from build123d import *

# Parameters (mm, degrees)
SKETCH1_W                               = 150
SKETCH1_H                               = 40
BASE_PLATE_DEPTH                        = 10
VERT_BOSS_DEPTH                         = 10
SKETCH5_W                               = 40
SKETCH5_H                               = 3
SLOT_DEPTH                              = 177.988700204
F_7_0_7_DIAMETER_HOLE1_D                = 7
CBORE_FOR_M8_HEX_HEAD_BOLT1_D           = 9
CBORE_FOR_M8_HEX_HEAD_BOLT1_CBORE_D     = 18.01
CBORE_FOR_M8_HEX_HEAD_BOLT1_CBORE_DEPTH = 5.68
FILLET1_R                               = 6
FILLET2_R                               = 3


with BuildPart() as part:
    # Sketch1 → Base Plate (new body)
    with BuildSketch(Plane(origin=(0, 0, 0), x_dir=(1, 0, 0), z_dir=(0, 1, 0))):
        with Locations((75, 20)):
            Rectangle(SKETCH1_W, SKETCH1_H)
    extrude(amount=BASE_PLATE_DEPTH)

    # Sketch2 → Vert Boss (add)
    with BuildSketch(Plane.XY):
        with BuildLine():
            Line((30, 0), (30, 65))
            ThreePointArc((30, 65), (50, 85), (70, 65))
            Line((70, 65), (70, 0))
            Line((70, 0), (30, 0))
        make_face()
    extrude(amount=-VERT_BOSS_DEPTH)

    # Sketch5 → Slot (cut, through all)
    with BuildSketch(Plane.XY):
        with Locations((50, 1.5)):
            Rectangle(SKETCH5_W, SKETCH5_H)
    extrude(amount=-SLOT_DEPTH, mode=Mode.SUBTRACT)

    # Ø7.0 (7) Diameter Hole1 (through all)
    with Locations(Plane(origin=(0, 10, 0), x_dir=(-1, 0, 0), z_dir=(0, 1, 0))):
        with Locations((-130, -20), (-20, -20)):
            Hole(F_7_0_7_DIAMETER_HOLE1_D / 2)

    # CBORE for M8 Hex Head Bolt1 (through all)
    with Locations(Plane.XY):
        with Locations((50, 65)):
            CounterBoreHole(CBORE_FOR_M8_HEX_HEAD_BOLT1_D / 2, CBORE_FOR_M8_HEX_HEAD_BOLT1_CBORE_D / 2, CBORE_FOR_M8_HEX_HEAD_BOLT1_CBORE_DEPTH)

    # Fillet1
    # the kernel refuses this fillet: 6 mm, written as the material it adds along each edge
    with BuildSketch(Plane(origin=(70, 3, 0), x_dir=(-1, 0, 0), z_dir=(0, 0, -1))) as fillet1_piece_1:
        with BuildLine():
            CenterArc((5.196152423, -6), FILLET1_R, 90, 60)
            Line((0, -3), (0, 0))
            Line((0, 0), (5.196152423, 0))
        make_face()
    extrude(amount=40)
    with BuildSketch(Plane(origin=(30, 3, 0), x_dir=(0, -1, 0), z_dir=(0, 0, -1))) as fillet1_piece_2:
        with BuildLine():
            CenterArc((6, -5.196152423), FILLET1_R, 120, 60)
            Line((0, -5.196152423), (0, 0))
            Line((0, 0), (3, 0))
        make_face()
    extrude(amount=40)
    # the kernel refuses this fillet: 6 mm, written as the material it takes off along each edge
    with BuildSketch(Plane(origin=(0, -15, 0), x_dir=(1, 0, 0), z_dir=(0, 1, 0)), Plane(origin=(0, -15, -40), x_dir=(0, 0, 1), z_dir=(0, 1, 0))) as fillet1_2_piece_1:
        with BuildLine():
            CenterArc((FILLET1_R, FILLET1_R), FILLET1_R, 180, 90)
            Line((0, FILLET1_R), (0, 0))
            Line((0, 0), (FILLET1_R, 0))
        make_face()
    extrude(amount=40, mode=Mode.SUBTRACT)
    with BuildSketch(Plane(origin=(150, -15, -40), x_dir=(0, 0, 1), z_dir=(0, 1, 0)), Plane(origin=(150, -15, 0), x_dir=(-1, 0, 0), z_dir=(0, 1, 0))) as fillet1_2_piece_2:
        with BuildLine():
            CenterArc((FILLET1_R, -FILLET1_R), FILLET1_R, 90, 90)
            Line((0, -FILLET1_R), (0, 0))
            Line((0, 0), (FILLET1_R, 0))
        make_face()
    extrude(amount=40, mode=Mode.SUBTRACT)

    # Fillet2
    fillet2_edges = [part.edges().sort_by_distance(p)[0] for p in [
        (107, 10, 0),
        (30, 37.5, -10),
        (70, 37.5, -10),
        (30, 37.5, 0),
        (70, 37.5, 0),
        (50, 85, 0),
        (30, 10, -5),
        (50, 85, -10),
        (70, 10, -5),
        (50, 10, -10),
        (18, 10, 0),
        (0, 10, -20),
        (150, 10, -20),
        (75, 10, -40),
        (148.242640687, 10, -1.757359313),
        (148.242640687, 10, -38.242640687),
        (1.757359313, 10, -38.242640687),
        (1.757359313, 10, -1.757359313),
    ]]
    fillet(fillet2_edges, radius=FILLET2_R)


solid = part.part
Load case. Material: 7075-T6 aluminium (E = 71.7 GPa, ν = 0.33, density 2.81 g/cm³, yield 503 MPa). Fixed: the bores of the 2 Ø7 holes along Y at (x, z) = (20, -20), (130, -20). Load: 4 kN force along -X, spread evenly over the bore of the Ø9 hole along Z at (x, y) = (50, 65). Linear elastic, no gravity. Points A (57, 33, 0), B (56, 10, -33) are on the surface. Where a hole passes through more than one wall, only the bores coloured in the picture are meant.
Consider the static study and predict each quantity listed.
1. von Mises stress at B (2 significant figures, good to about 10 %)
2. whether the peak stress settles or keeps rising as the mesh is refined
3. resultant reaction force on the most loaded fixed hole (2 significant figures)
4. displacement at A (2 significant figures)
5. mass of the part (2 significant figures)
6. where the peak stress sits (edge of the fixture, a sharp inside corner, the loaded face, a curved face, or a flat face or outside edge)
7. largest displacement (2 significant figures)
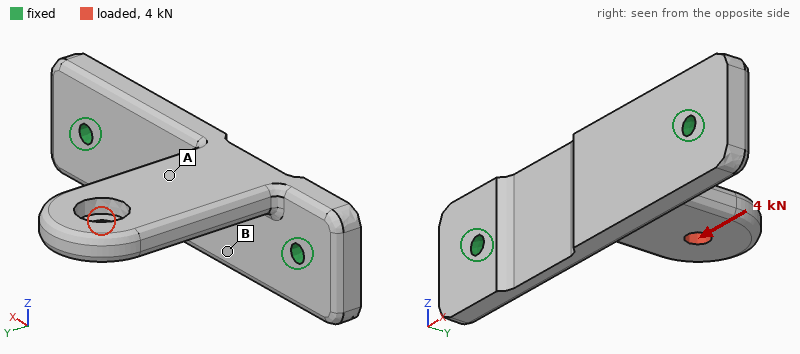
61 MPa
keeps rising
3.3 kN
0.32 mm
220 g
a sharp inside corner
0.80 mm
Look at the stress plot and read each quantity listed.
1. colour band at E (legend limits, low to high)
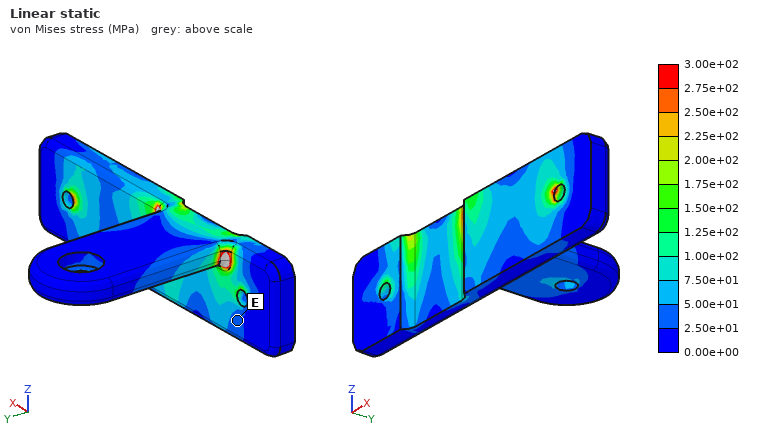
2.50e+01 to 5.00e+01 MPa
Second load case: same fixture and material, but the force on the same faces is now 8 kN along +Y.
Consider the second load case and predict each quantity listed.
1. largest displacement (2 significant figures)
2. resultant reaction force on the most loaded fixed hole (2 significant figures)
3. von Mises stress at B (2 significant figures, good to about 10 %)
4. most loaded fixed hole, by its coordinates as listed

0.44 mm
6.4 kN
55 MPa
(20, -20)
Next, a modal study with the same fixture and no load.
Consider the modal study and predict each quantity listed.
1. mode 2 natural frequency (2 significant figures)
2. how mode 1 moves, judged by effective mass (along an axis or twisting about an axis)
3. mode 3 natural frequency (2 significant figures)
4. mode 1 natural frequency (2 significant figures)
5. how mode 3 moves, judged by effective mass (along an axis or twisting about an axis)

1900 Hz
along Z
4500 Hz
1100 Hz
along Y
